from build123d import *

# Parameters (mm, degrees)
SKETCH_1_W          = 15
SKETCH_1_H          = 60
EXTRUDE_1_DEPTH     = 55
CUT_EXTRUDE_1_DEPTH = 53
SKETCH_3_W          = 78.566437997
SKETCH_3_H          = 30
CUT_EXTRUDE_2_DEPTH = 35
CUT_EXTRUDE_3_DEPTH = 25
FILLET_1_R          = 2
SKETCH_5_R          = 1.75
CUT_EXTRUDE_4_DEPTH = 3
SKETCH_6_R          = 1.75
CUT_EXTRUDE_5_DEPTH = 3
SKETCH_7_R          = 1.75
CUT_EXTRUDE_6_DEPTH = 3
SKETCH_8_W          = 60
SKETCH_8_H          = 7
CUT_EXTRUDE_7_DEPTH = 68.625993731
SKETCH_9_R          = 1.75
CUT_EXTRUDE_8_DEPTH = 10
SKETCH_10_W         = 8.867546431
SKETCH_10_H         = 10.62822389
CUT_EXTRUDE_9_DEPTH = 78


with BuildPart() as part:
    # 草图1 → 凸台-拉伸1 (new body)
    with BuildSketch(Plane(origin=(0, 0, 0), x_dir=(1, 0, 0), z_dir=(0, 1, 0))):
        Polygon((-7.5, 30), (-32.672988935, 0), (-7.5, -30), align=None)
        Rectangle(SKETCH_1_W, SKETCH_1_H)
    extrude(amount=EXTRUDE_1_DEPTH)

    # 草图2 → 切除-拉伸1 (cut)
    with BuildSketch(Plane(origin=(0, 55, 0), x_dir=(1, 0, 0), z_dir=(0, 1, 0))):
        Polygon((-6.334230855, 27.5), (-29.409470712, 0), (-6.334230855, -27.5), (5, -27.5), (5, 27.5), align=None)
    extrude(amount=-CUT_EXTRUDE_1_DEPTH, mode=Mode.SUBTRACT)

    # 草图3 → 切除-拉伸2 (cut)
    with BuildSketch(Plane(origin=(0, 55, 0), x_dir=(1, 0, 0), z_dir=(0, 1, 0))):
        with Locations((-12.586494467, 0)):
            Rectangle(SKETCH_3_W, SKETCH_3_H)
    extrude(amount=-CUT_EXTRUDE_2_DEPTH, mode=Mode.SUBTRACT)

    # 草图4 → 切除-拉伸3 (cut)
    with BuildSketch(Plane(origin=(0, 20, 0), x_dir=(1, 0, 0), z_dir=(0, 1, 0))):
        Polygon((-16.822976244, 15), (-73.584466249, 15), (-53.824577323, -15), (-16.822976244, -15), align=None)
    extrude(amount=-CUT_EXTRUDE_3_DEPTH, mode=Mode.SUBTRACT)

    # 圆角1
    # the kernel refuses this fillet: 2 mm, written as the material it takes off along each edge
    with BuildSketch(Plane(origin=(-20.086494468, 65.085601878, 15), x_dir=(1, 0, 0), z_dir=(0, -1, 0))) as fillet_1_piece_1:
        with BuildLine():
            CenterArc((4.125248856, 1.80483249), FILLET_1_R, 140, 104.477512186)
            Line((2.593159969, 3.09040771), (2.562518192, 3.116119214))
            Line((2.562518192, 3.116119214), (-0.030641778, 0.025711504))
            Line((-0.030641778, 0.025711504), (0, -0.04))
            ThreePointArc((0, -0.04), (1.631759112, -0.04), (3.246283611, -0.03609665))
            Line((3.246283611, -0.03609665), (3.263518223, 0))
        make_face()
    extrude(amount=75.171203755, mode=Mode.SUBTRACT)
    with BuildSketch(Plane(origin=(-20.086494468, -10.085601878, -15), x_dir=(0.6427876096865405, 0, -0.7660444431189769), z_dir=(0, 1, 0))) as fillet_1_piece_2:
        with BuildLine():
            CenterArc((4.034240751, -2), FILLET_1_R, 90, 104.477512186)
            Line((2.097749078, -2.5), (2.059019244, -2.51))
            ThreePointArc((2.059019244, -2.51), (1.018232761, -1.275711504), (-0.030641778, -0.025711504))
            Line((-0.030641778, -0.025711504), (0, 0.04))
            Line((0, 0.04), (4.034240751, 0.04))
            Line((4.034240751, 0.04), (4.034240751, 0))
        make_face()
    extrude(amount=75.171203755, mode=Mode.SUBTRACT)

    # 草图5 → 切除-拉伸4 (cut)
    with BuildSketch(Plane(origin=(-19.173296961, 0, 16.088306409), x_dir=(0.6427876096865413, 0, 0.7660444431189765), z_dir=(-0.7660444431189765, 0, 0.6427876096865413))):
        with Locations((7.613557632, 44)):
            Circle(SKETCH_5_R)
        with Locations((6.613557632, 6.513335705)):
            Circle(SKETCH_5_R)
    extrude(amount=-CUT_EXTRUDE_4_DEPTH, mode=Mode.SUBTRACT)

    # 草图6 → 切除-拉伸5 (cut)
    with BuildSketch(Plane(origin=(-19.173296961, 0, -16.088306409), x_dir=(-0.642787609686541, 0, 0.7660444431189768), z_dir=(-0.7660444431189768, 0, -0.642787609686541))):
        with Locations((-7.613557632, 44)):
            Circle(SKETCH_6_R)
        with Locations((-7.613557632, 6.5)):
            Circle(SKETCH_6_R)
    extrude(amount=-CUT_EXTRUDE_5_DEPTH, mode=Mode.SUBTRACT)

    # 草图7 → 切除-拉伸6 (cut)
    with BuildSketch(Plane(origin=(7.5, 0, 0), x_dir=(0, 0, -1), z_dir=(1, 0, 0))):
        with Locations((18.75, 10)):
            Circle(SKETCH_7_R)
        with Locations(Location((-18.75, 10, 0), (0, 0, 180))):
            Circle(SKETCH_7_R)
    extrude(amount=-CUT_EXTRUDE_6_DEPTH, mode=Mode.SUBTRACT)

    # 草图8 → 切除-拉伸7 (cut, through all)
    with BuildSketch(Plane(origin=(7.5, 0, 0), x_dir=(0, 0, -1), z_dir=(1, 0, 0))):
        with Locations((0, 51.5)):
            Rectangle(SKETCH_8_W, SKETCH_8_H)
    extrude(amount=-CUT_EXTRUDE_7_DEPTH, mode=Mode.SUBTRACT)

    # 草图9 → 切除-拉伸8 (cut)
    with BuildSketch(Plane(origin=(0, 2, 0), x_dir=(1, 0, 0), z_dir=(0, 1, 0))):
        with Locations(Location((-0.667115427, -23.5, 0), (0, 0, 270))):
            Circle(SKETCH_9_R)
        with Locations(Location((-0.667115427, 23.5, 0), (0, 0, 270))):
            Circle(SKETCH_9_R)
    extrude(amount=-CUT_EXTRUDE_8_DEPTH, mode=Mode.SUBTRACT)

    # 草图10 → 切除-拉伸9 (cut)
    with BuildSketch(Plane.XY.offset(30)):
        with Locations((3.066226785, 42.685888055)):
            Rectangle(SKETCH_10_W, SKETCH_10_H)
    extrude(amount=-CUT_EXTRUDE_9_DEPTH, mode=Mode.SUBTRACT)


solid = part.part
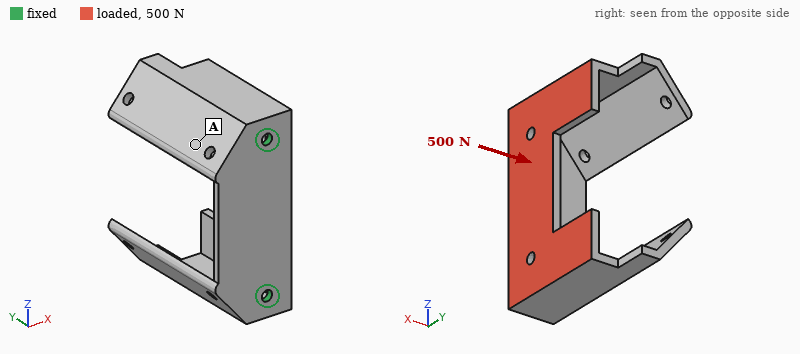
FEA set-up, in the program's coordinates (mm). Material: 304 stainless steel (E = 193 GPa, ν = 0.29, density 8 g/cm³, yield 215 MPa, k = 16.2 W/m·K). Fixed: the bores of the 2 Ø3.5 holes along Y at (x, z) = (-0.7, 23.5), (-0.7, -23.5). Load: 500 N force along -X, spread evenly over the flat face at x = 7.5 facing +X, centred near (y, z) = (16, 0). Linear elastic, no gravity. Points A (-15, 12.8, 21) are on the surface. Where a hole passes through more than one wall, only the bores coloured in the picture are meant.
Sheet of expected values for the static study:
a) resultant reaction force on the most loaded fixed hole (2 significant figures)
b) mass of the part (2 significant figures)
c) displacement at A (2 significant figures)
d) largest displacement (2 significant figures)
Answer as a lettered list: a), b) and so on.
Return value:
a) 250 N
b) 100 g
c) 0.042 mm
d) 0.13 mm
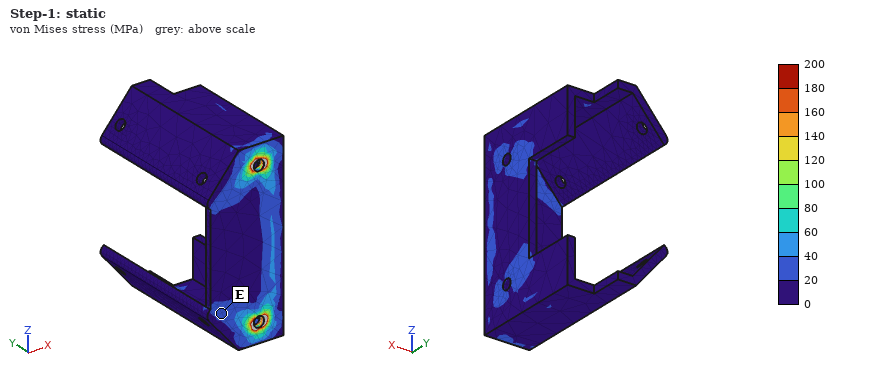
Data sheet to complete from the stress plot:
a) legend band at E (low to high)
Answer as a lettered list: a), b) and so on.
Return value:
a) 20 to 40 MPa
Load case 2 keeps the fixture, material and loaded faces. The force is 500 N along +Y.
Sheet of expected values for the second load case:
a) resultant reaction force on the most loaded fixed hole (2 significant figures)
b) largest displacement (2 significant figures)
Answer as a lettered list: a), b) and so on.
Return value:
a) 260 N
b) 57 µm
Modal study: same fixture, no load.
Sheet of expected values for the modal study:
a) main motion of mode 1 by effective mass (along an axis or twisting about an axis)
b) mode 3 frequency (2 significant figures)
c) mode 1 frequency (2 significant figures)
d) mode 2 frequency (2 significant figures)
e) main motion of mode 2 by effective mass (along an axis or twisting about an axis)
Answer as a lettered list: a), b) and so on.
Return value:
a) along X
b) 2100 Hz
c) 1200 Hz
d) 1500 Hz
e) twisting about Y
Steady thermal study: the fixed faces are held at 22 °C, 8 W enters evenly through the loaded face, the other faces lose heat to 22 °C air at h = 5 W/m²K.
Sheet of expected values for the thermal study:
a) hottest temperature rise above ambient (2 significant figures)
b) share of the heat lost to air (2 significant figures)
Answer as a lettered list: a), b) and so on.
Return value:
a) 56 K
b) 21 %
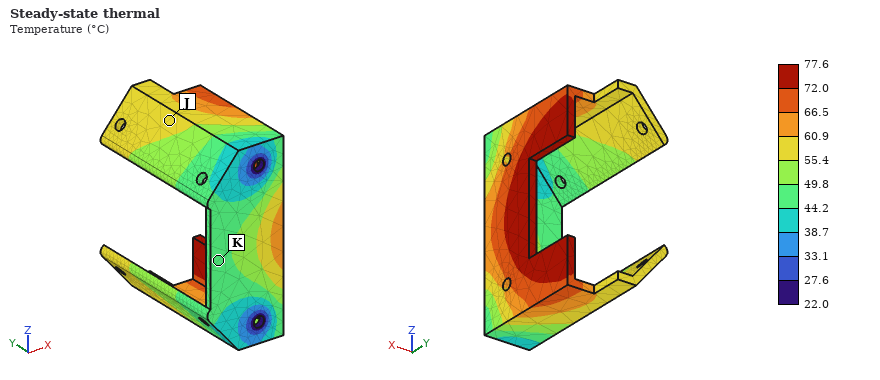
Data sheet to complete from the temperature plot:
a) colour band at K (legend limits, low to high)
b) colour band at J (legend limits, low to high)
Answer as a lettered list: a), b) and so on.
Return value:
a) 44.2 to 49.8 °C
b) 55.4 to 60.9 °C
